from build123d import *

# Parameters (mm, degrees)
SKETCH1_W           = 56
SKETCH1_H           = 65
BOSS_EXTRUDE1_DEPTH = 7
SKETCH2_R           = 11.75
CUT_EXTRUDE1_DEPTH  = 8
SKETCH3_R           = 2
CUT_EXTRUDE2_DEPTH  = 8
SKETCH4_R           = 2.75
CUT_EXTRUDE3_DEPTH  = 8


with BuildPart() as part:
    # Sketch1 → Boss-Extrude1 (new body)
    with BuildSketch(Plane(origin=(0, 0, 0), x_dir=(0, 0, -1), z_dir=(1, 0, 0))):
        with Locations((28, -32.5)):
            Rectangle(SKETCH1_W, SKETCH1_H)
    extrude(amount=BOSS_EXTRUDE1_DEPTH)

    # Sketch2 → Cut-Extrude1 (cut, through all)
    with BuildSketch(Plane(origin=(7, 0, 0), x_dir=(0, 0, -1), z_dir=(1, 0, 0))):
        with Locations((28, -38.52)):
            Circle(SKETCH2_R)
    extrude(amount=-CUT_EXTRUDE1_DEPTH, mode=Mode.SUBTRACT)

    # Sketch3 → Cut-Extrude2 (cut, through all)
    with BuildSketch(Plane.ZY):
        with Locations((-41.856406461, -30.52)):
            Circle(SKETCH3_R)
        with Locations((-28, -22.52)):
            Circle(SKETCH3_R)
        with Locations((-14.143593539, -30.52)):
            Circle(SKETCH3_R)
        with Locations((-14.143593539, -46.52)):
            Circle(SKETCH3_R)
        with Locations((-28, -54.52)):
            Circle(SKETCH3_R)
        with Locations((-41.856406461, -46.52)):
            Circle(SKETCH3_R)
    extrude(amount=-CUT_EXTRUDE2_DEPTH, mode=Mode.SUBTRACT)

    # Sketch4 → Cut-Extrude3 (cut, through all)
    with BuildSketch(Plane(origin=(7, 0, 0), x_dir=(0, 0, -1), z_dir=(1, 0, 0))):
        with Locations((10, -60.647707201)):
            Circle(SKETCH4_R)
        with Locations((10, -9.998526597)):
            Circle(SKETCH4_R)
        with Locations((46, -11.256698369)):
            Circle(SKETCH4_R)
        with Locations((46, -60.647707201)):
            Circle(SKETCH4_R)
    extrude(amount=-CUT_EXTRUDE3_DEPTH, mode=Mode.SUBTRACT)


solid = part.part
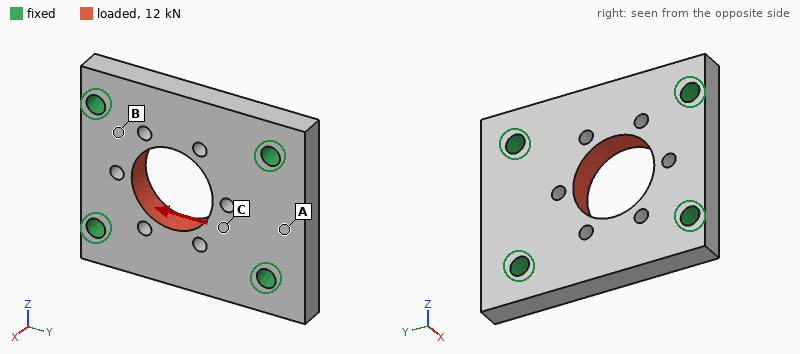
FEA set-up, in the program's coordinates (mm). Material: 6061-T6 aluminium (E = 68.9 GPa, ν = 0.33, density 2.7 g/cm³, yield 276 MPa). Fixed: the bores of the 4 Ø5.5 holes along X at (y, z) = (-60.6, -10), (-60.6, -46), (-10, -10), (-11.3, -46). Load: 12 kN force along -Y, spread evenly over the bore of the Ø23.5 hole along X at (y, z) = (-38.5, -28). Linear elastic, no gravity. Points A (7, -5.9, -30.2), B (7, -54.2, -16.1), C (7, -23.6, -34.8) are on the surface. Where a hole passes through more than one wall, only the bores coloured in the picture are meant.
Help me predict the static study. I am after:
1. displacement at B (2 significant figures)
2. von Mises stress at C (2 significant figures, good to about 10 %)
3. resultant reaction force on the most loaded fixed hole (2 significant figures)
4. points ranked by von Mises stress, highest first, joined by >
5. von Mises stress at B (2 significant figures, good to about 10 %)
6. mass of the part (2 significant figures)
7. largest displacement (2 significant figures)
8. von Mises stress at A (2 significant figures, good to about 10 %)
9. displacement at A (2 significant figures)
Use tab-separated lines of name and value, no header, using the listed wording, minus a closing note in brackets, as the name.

displacement at B	5.5 µm
von Mises stress at C	21 MPa
resultant reaction force on the most loaded fixed hole	3.3 kN
points ranked by von Mises stress, highest first, joined by >	B > C > A
von Mises stress at B	38 MPa
mass of the part	57 g
largest displacement	15 µm
von Mises stress at A	6.0 MPa
displacement at A	5.0 µm
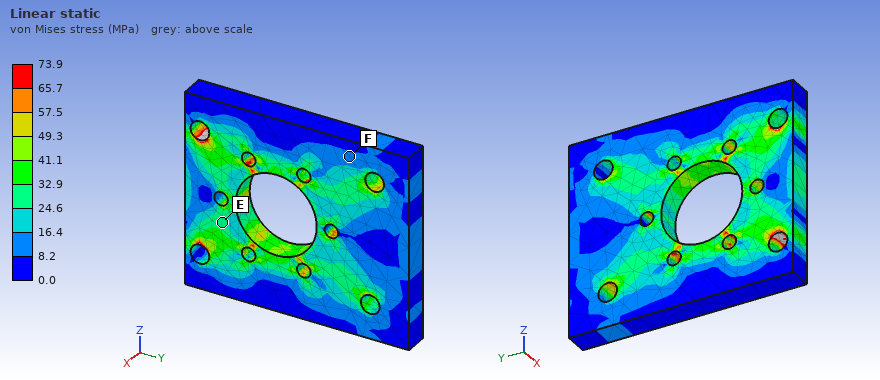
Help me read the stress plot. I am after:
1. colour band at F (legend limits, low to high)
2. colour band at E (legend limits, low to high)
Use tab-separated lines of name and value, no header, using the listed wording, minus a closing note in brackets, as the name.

colour band at F	8.2 to 16.4 MPa
colour band at E	24.6 to 32.9 MPa
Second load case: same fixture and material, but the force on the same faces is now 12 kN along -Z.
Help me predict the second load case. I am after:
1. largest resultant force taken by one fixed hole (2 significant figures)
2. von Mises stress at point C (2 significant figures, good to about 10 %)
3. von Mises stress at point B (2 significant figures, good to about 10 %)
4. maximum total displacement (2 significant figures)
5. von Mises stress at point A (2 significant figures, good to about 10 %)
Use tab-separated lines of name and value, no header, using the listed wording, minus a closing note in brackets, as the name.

largest resultant force taken by one fixed hole	3.3 kN
von Mises stress at point C	37 MPa
von Mises stress at point B	35 MPa
maximum total displacement	21 µm
von Mises stress at point A	8.0 MPa
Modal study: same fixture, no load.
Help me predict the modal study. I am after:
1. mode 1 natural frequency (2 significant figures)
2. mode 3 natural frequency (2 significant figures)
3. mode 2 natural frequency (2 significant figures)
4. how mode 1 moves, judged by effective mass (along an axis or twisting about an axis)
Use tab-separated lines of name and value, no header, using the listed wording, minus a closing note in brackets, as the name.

mode 1 natural frequency	13 kHz
mode 3 natural frequency	19 kHz
mode 2 natural frequency	15 kHz
how mode 1 moves, judged by effective mass	along X
